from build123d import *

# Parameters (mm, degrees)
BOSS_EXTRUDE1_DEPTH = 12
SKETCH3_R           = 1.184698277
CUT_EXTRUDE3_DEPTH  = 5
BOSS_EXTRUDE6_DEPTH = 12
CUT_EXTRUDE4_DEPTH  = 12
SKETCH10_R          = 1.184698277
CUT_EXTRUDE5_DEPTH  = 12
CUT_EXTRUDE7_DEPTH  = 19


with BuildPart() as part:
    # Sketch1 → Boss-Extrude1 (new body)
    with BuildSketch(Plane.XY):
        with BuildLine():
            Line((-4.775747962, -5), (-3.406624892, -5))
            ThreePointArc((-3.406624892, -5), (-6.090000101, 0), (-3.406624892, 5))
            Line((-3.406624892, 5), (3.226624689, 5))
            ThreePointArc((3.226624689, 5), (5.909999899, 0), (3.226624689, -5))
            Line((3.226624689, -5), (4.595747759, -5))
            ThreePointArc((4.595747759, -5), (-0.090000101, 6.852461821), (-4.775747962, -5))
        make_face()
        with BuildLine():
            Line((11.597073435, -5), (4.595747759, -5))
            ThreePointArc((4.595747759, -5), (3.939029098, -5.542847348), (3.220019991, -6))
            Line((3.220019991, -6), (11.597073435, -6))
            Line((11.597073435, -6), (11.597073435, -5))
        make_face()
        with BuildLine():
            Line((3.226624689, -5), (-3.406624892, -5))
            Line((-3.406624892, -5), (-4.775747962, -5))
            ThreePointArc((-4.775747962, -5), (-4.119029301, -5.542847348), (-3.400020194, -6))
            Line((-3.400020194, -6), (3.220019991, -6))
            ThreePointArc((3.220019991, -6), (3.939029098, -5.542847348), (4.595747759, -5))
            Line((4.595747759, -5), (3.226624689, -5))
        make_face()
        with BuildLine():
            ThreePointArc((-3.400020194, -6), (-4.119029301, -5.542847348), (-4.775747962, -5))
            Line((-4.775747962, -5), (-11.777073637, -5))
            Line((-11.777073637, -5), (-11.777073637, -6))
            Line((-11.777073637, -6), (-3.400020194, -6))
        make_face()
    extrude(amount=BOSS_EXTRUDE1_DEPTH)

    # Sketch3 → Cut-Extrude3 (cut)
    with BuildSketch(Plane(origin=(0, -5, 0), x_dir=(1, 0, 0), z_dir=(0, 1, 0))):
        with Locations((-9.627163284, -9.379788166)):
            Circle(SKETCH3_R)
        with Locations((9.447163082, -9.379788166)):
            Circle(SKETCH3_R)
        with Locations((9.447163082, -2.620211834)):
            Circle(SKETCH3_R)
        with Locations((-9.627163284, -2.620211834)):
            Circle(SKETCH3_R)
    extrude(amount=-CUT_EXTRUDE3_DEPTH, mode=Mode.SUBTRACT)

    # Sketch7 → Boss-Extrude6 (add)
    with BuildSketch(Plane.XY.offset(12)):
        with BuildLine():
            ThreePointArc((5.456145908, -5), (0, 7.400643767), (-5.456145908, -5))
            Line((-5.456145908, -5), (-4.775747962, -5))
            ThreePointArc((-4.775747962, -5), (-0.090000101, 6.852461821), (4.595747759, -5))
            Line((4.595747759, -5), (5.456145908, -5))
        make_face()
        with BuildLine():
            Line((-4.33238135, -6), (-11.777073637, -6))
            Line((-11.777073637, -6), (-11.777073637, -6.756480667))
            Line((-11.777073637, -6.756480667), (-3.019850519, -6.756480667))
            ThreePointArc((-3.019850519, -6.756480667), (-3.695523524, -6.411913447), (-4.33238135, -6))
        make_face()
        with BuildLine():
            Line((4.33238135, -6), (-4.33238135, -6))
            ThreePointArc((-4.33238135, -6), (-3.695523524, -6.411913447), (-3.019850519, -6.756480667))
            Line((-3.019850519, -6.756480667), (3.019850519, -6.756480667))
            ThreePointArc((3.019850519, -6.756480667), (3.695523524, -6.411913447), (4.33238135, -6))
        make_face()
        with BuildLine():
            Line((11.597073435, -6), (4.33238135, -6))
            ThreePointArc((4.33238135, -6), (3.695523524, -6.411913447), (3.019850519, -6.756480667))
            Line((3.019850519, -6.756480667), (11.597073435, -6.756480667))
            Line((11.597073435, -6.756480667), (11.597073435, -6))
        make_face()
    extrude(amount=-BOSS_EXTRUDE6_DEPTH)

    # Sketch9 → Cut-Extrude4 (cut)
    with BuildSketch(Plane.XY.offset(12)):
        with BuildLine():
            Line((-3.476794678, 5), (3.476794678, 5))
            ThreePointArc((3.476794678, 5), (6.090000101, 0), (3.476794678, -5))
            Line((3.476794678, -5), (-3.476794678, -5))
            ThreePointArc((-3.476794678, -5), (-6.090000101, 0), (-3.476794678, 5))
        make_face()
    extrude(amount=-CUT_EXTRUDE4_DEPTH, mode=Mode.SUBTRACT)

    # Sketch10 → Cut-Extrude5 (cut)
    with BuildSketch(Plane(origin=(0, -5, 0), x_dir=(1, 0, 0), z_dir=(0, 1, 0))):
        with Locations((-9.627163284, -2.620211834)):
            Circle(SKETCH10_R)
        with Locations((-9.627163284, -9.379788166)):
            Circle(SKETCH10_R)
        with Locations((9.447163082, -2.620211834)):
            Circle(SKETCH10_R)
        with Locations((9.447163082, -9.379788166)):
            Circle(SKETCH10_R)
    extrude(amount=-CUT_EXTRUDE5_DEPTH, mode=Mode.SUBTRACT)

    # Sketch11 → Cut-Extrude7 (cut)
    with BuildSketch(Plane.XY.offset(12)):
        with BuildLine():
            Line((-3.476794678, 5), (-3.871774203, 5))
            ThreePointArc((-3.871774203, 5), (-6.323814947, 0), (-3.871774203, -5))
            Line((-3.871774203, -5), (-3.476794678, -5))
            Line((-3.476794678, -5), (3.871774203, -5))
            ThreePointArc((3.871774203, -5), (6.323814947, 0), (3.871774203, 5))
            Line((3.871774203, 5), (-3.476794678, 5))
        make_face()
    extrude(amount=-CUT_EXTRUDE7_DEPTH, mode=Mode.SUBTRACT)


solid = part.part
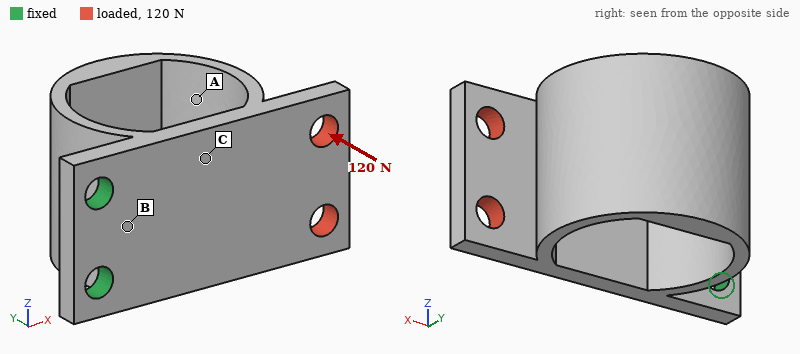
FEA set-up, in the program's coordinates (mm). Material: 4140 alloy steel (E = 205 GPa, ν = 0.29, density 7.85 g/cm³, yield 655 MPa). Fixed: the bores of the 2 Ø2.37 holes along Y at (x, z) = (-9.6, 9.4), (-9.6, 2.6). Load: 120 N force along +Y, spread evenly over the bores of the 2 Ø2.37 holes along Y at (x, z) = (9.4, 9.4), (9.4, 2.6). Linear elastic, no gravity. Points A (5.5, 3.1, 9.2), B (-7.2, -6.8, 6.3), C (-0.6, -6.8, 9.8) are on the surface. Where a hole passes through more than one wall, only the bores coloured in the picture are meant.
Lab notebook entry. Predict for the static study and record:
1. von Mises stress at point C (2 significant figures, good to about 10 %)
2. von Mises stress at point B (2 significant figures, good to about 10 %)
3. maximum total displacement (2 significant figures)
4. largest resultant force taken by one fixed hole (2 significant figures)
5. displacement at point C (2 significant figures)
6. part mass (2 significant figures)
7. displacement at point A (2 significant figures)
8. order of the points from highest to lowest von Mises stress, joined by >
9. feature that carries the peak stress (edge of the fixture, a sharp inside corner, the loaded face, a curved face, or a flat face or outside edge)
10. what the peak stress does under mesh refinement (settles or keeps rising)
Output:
140 MPa
260 MPa
0.22 mm
61 N
0.054 mm
7.6 g
0.16 mm
B > C > A
edge of the fixture
keeps rising
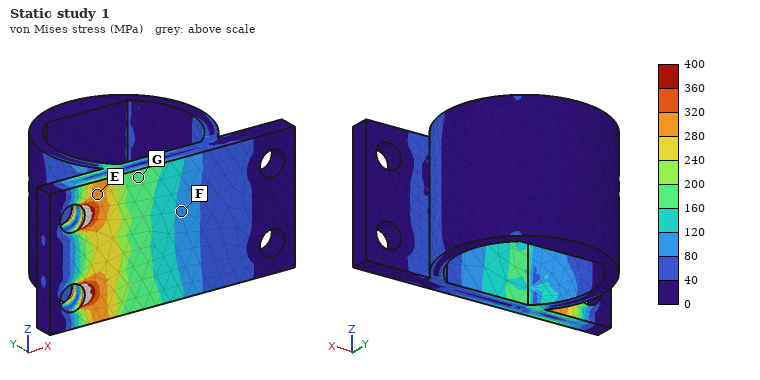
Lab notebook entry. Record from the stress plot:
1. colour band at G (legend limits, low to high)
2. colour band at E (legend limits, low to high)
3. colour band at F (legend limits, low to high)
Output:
160 to 200 MPa
280 to 320 MPa
80 to 120 MPa
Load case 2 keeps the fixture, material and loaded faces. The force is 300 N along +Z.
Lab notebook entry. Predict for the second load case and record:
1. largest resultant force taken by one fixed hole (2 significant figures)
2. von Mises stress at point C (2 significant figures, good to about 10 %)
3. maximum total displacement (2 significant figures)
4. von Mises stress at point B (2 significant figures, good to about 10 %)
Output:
700 N
50 MPa
21 µm
37 MPa
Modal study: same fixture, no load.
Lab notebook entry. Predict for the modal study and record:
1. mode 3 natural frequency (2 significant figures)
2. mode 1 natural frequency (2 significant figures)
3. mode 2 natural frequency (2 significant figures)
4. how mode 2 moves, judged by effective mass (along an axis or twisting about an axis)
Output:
8100 Hz
2200 Hz
5900 Hz
along Z
